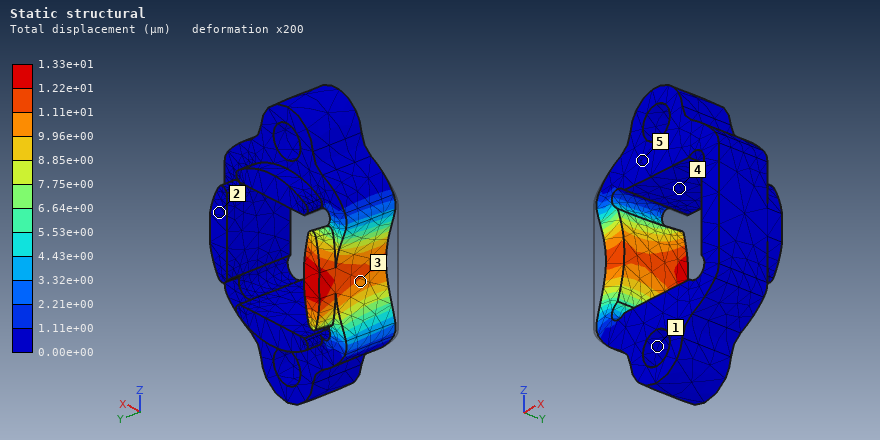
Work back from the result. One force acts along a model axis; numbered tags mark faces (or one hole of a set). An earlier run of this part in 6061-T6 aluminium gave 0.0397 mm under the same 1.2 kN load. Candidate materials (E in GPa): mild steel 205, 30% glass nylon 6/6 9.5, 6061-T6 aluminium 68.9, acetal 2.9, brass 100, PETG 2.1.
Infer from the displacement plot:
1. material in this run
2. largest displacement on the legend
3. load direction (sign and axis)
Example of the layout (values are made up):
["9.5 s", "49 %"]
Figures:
["mild steel", "1.33e+01 µm", "+X"]
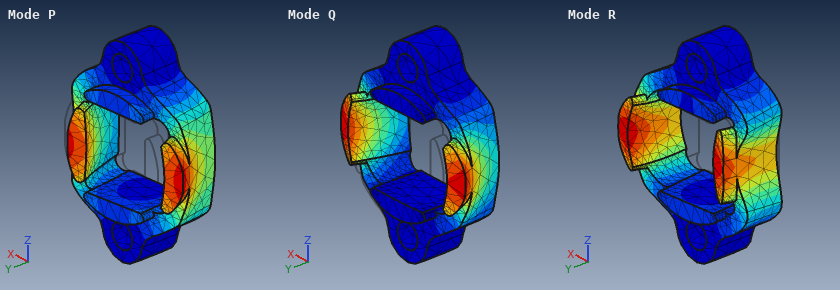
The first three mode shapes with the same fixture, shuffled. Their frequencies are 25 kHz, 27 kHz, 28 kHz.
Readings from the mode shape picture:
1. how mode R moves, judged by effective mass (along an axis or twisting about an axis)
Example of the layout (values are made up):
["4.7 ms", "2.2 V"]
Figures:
["along X"]
